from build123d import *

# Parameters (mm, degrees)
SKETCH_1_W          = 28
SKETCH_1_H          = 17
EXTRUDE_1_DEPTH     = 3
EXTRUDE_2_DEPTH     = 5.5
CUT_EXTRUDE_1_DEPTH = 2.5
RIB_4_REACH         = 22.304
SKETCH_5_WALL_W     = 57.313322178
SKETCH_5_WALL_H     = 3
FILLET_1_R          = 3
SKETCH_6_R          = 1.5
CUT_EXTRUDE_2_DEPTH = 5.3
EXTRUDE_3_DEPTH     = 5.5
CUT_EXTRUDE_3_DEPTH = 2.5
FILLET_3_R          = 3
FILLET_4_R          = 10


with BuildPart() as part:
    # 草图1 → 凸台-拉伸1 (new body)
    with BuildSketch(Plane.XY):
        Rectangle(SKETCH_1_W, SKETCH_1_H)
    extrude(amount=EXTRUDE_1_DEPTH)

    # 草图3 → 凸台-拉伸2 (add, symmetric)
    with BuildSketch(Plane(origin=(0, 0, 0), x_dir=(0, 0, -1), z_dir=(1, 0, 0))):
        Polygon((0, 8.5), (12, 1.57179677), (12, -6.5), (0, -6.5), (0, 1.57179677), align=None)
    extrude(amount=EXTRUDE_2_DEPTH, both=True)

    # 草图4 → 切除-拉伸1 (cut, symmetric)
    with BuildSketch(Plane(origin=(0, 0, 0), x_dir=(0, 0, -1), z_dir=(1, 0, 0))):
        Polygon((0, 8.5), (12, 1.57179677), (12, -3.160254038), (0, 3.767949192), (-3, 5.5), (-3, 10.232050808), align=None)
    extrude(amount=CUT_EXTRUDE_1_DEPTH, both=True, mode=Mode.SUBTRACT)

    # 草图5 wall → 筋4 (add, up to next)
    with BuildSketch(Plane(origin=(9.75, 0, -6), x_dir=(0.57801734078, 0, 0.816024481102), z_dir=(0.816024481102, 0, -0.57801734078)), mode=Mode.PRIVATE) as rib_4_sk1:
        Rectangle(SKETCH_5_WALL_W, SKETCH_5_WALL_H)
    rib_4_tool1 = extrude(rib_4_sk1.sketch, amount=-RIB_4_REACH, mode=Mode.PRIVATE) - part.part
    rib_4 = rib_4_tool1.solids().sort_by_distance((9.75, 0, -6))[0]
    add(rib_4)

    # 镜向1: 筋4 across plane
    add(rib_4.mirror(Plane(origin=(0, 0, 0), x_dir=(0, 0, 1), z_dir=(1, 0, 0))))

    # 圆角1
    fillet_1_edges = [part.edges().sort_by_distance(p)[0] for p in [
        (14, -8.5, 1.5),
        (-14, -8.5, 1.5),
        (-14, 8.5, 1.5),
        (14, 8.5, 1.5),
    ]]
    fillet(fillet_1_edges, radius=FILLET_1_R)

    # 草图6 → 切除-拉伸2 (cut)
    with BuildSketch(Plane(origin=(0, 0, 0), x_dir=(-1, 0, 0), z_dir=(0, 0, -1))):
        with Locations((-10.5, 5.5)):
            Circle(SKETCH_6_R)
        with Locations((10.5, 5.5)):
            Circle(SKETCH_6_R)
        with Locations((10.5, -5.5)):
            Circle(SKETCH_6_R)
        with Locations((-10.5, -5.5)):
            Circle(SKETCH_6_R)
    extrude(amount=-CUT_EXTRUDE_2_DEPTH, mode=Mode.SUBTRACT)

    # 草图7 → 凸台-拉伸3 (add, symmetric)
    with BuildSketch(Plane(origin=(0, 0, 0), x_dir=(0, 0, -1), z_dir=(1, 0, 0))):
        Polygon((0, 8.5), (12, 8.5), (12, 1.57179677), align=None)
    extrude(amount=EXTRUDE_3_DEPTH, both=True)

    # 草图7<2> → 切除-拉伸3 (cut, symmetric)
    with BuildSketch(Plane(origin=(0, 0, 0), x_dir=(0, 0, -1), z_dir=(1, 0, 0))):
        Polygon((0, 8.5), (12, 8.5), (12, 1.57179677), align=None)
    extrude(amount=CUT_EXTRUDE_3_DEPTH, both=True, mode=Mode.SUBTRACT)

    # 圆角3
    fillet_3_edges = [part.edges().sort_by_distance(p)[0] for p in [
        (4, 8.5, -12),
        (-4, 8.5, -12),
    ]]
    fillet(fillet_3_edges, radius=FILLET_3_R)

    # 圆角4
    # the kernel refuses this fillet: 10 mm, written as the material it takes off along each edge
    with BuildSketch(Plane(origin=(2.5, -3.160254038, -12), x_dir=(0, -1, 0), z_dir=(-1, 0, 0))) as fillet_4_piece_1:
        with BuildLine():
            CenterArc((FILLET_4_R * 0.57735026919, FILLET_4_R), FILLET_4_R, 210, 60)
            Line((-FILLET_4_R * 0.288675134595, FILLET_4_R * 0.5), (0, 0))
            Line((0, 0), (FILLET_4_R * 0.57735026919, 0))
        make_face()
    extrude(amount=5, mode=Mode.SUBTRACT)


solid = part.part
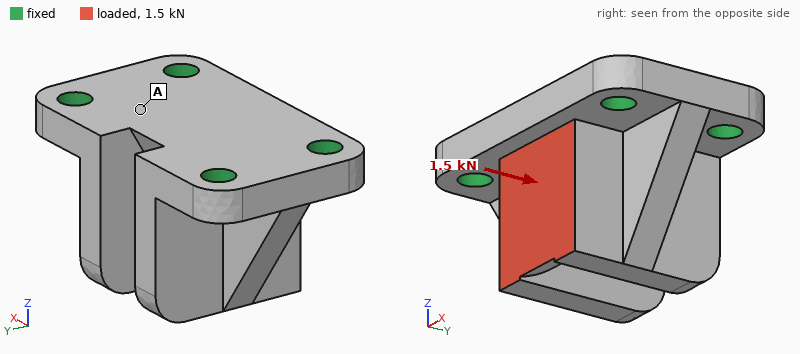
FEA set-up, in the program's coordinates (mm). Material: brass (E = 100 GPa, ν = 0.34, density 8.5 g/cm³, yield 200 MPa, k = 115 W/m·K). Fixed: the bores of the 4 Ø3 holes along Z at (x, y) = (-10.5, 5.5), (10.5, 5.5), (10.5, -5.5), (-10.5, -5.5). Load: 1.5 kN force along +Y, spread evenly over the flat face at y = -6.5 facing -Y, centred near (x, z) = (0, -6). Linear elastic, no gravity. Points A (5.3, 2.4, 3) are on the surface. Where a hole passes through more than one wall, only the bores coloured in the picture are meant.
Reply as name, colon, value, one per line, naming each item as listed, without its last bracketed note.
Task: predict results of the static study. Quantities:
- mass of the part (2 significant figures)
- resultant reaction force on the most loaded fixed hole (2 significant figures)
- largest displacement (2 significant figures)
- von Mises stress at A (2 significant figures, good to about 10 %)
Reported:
mass of the part: 26 g
resultant reaction force on the most loaded fixed hole: 720 N
largest displacement: 26 µm
von Mises stress at A: 20 MPa
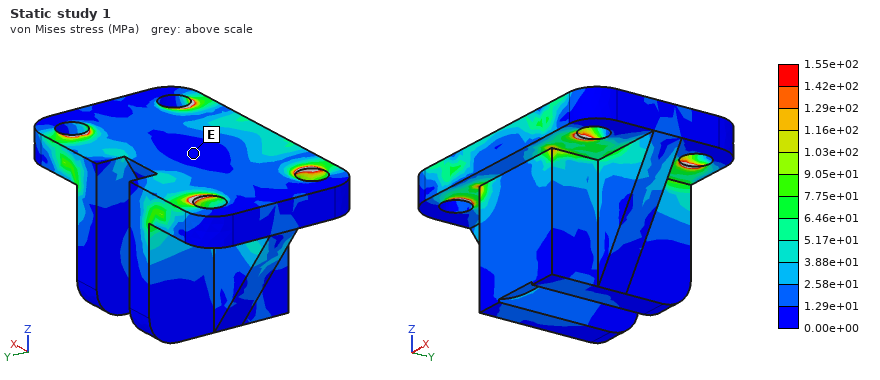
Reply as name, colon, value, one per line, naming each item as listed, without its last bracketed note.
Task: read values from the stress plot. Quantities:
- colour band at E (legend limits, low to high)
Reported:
colour band at E: 0.00e+00 to 1.29e+01 MPa
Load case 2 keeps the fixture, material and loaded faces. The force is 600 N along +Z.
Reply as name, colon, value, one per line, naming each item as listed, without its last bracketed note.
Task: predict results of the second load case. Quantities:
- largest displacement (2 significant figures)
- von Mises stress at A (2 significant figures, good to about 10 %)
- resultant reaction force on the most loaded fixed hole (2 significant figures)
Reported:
largest displacement: 10 µm
von Mises stress at A: 12 MPa
resultant reaction force on the most loaded fixed hole: 340 N
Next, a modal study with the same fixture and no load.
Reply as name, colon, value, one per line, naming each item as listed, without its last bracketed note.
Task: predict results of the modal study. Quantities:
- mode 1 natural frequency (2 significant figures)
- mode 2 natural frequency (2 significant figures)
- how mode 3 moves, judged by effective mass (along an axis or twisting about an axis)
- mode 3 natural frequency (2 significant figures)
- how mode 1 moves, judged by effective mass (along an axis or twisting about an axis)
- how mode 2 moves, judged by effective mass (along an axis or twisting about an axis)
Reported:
mode 1 natural frequency: 12 kHz
mode 2 natural frequency: 19 kHz
how mode 3 moves, judged by effective mass: along X
mode 3 natural frequency: 20 kHz
how mode 1 moves, judged by effective mass: along Y
how mode 2 moves, judged by effective mass: along Z
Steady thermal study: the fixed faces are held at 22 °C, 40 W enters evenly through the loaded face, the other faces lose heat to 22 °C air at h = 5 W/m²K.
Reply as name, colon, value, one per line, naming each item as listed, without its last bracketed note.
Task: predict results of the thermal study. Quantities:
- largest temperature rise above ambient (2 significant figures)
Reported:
largest temperature rise above ambient: 45 K
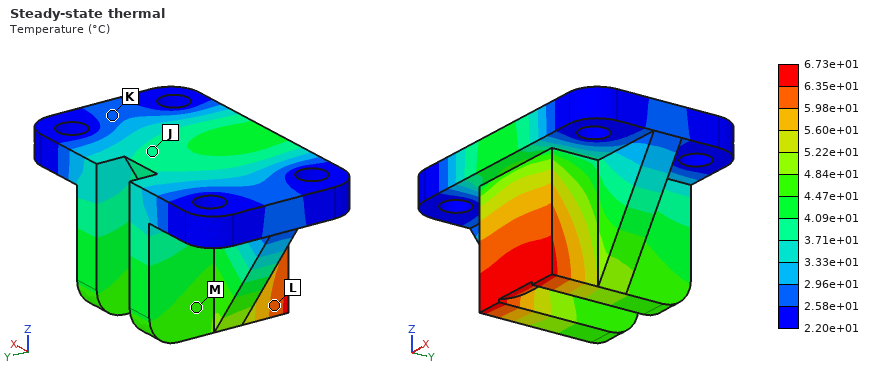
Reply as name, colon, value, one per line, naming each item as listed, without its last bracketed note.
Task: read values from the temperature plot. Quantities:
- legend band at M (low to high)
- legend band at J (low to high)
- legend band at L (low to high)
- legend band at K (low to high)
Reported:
legend band at M: 4.47e+01 to 4.84e+01 °C
legend band at J: 3.71e+01 to 4.09e+01 °C
legend band at L: 5.98e+01 to 6.35e+01 °C
legend band at K: 2.58e+01 to 2.96e+01 °C
